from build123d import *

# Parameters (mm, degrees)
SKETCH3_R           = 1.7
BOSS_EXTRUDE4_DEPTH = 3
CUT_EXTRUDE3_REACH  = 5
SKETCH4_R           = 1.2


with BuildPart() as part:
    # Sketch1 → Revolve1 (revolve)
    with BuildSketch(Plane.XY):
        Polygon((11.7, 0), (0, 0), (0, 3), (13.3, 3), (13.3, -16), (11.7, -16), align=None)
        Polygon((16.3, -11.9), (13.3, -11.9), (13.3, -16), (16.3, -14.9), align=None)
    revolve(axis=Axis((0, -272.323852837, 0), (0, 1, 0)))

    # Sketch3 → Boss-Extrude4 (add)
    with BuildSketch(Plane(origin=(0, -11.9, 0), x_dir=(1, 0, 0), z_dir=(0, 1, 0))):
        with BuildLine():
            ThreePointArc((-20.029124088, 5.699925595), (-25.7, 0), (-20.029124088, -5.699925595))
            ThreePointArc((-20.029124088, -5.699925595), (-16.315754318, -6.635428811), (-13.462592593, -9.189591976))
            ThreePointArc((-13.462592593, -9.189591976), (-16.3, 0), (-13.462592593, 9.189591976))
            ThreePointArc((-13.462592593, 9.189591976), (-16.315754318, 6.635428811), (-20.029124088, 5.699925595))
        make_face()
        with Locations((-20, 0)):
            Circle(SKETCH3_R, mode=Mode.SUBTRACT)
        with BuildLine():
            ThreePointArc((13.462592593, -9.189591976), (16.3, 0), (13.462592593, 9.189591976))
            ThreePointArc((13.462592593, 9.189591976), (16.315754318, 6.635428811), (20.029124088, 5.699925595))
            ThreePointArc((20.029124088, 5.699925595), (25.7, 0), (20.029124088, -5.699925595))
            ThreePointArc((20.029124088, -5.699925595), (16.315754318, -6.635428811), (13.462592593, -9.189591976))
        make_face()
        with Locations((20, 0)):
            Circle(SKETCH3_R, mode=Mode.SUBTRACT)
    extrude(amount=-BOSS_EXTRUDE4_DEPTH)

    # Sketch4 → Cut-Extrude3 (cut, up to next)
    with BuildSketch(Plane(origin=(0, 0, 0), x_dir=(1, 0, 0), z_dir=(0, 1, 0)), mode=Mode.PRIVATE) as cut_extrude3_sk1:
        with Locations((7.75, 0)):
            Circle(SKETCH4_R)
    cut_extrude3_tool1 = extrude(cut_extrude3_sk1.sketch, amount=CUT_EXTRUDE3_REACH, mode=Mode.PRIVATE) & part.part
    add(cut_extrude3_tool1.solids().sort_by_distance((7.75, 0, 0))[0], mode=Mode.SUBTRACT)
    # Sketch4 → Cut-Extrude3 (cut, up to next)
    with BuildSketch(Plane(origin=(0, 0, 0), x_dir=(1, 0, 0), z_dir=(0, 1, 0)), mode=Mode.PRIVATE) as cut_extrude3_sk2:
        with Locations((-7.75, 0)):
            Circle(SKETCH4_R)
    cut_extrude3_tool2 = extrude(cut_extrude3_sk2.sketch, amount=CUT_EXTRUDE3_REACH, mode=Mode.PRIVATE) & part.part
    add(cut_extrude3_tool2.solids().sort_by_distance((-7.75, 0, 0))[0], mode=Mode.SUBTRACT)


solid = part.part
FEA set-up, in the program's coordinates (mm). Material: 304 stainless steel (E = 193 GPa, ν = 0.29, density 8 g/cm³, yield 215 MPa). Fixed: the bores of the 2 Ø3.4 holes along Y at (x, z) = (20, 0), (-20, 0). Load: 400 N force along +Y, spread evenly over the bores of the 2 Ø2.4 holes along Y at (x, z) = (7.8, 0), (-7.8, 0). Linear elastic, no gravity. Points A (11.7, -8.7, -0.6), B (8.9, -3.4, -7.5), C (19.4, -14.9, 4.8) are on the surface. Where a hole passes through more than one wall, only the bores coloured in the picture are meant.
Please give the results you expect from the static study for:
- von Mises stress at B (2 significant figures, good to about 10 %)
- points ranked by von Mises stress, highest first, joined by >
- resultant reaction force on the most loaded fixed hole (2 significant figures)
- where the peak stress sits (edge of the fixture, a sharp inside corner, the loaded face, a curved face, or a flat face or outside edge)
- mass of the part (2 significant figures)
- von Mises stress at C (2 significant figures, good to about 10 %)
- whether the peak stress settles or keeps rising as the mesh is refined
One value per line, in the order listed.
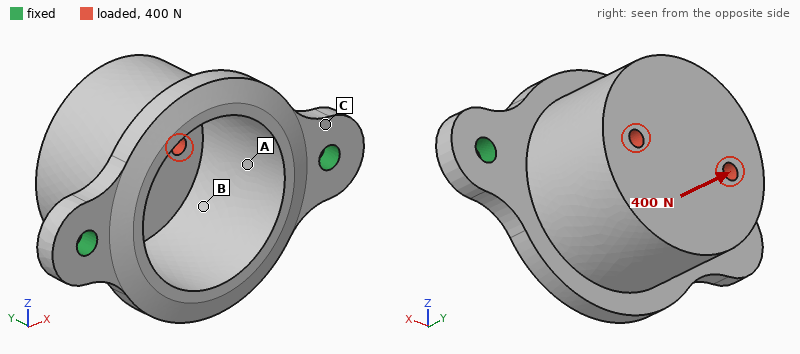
9.8 MPa
C > B > A
210 N
edge of the fixture
42 g
17 MPa
keeps rising
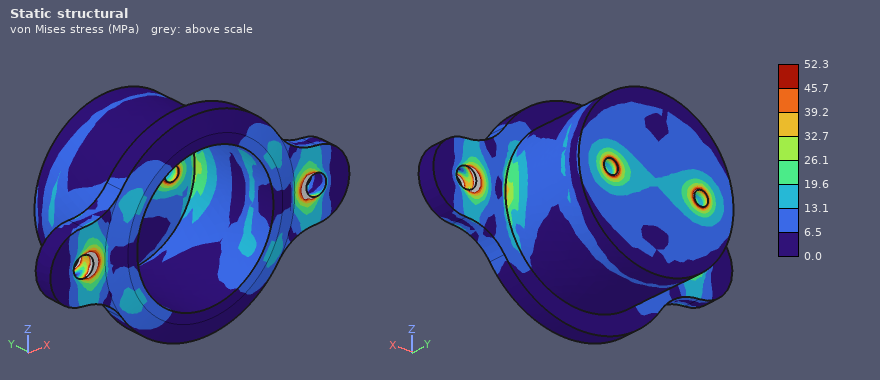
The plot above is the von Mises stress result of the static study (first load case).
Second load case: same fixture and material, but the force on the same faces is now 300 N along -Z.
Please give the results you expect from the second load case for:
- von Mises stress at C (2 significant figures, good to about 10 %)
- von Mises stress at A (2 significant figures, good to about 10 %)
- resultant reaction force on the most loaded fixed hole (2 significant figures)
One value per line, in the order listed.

53 MPa
22 MPa
150 N
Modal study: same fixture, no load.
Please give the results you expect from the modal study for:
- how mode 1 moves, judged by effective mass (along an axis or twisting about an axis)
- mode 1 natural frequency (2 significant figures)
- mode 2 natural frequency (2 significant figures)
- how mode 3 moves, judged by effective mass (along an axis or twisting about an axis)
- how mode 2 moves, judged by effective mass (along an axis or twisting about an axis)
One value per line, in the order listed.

along Z
3200 Hz
9100 Hz
along X
along Y
